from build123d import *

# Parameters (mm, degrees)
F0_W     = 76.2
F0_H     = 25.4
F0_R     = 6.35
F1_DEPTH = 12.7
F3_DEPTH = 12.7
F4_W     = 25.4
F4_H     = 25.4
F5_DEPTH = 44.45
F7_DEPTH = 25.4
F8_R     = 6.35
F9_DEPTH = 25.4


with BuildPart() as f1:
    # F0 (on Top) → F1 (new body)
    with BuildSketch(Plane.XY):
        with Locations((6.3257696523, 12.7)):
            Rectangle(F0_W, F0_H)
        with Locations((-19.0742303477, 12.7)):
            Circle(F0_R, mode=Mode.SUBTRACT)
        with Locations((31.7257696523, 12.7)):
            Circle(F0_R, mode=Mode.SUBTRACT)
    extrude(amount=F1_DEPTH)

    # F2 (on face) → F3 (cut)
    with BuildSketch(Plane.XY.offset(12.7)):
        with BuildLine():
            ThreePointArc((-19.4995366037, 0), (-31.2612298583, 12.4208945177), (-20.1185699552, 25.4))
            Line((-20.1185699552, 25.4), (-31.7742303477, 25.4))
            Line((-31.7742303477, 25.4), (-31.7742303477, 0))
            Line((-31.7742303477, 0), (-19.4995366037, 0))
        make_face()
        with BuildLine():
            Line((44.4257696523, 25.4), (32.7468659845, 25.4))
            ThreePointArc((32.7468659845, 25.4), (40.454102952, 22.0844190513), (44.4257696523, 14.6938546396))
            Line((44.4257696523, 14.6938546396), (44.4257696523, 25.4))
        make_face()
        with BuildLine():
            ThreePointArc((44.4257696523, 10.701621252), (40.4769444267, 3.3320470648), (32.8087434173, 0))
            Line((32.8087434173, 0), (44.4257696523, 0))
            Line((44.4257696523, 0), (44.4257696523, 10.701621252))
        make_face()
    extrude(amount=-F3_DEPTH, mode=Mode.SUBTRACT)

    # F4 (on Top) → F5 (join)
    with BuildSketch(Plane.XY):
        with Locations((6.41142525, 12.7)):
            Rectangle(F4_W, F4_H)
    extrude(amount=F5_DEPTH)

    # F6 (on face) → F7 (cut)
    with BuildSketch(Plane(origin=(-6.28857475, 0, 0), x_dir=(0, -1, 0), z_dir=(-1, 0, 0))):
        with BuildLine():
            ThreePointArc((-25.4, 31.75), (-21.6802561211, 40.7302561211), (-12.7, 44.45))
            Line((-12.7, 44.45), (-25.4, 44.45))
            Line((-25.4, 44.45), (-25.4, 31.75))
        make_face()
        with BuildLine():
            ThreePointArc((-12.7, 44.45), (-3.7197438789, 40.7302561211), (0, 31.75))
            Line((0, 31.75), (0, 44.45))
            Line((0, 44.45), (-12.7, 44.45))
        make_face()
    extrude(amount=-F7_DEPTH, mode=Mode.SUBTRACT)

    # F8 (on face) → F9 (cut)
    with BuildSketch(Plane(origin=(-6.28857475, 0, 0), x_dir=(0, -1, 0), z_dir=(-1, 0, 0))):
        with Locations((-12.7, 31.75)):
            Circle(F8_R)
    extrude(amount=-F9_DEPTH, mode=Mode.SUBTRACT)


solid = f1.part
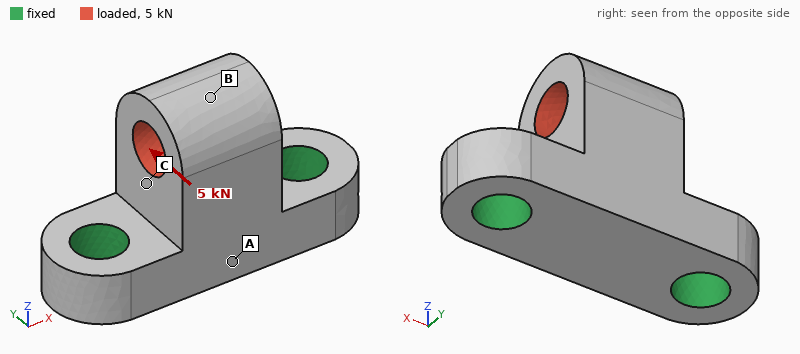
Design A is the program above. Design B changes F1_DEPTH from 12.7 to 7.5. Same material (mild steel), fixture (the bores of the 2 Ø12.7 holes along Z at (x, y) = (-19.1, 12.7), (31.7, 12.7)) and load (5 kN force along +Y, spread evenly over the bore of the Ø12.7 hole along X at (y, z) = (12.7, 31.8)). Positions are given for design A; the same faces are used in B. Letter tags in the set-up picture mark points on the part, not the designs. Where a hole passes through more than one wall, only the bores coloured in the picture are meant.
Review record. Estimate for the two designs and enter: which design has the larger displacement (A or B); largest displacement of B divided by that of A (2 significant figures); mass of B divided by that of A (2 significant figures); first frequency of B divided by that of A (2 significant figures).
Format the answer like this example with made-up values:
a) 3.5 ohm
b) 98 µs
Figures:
a) B
b) 2.7
c) 0.87
d) 0.60
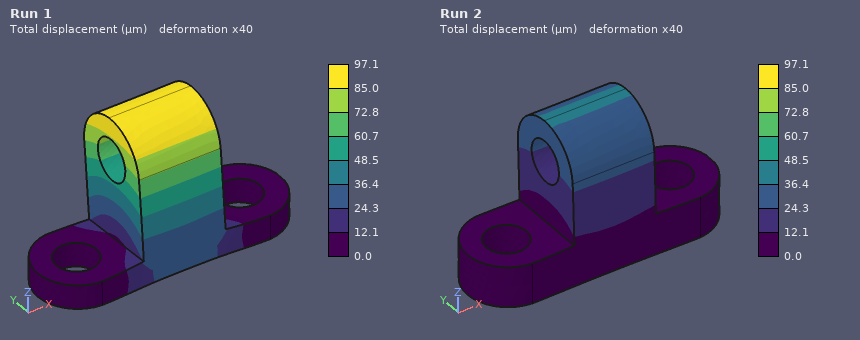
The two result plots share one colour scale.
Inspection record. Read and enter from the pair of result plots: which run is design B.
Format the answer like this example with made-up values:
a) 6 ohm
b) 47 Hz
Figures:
a) Run 1
